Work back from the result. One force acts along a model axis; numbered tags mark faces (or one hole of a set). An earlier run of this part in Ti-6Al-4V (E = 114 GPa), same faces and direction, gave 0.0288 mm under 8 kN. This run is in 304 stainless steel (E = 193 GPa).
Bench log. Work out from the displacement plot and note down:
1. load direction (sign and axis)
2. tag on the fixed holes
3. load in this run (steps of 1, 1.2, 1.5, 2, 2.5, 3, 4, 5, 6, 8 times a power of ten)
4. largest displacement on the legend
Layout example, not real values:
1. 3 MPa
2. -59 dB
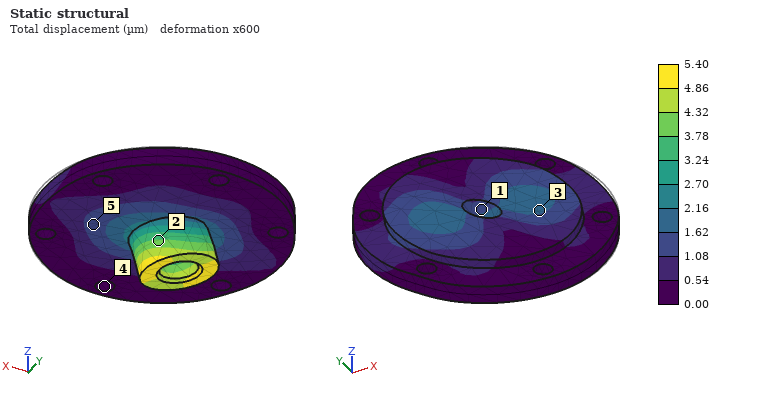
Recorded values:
1. -X
2. 4
3. 2.5 kN
4. 5.40 µm
